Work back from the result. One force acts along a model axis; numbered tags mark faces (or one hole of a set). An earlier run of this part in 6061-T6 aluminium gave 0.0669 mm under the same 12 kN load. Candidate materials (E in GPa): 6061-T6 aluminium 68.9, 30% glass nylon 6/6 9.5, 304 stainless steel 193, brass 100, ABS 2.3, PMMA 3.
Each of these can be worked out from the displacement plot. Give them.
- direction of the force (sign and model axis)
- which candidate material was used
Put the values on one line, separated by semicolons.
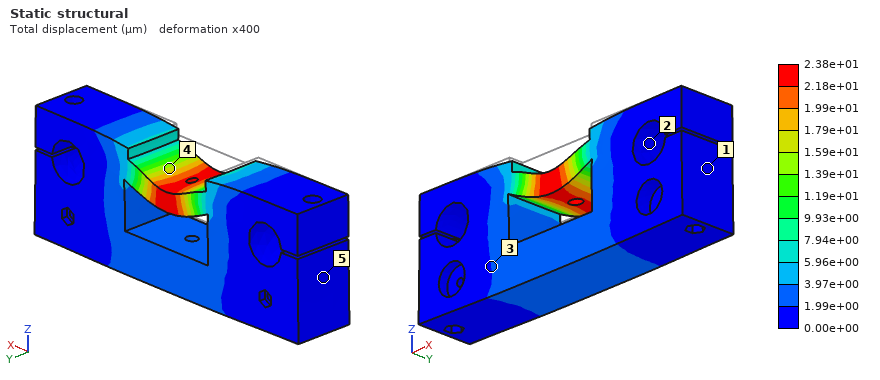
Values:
-Z; 304 stainless steel
